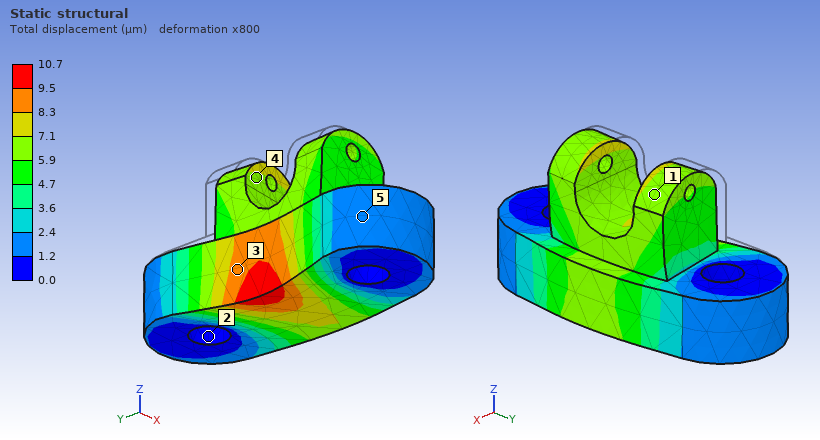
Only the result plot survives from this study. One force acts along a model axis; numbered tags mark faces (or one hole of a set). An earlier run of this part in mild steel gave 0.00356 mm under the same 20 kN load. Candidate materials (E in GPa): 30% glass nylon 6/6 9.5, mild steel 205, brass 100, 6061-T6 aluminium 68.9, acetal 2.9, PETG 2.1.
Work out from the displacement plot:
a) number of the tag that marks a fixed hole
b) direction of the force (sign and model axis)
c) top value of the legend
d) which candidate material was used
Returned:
2
+X
10.7 µm
6061-T6 aluminium
